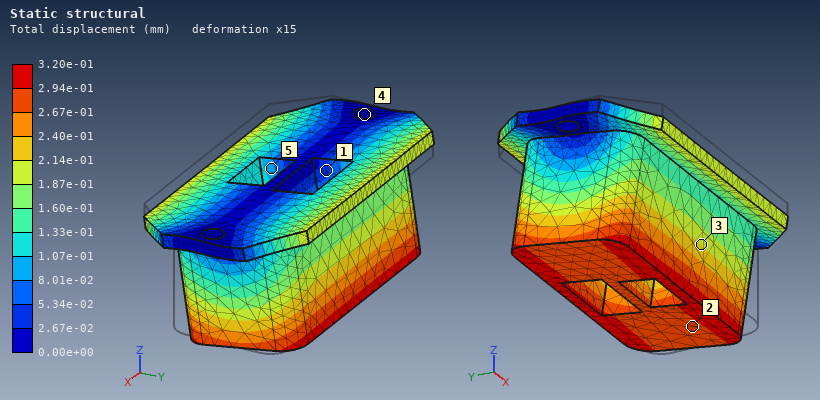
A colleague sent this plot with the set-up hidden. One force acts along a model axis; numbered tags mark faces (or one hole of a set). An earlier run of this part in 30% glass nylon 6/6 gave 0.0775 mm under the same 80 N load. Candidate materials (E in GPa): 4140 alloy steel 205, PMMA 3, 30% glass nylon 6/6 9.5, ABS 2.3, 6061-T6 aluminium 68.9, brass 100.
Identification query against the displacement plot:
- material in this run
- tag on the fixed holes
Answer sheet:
ABS
4
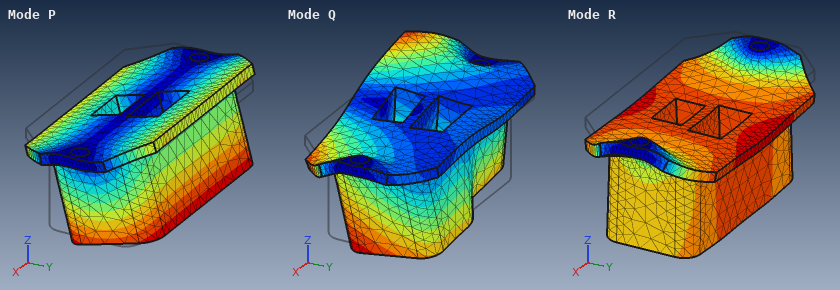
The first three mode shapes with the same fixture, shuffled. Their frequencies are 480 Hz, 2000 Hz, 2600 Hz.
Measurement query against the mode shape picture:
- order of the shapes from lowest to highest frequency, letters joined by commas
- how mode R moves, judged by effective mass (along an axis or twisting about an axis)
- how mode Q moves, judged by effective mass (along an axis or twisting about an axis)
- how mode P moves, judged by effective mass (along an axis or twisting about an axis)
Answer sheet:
P, R, Q
along Z
along X
along Y
